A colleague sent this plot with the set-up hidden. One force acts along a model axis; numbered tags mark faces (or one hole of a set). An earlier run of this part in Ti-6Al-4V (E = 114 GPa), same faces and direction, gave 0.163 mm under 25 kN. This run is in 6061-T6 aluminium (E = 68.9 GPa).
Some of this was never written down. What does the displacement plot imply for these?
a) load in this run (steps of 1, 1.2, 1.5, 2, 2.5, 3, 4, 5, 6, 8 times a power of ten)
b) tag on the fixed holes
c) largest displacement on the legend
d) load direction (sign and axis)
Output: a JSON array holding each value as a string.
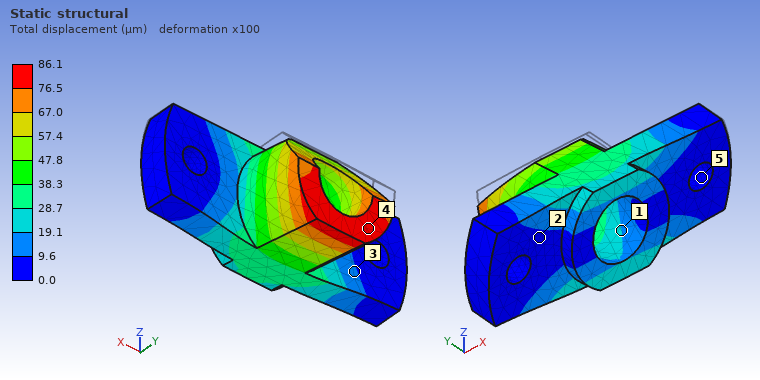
["8 kN", "5", "86.1 µm", "-Z"]
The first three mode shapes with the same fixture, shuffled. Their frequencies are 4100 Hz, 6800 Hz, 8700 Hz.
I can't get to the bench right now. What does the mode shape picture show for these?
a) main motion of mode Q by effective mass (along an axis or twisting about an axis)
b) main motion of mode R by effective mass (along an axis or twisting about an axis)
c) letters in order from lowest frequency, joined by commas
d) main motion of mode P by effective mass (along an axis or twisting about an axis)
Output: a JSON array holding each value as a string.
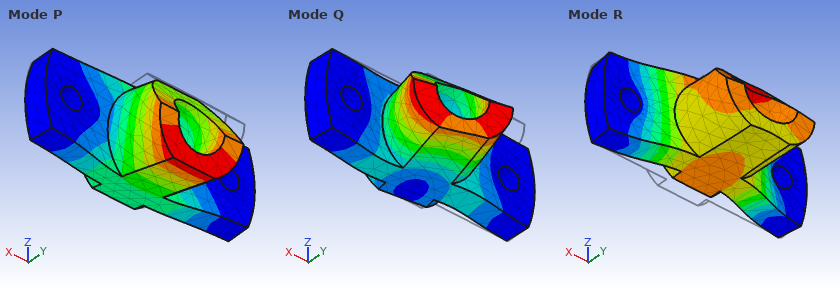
["along X", "along Y", "P, R, Q", "along Z"]
